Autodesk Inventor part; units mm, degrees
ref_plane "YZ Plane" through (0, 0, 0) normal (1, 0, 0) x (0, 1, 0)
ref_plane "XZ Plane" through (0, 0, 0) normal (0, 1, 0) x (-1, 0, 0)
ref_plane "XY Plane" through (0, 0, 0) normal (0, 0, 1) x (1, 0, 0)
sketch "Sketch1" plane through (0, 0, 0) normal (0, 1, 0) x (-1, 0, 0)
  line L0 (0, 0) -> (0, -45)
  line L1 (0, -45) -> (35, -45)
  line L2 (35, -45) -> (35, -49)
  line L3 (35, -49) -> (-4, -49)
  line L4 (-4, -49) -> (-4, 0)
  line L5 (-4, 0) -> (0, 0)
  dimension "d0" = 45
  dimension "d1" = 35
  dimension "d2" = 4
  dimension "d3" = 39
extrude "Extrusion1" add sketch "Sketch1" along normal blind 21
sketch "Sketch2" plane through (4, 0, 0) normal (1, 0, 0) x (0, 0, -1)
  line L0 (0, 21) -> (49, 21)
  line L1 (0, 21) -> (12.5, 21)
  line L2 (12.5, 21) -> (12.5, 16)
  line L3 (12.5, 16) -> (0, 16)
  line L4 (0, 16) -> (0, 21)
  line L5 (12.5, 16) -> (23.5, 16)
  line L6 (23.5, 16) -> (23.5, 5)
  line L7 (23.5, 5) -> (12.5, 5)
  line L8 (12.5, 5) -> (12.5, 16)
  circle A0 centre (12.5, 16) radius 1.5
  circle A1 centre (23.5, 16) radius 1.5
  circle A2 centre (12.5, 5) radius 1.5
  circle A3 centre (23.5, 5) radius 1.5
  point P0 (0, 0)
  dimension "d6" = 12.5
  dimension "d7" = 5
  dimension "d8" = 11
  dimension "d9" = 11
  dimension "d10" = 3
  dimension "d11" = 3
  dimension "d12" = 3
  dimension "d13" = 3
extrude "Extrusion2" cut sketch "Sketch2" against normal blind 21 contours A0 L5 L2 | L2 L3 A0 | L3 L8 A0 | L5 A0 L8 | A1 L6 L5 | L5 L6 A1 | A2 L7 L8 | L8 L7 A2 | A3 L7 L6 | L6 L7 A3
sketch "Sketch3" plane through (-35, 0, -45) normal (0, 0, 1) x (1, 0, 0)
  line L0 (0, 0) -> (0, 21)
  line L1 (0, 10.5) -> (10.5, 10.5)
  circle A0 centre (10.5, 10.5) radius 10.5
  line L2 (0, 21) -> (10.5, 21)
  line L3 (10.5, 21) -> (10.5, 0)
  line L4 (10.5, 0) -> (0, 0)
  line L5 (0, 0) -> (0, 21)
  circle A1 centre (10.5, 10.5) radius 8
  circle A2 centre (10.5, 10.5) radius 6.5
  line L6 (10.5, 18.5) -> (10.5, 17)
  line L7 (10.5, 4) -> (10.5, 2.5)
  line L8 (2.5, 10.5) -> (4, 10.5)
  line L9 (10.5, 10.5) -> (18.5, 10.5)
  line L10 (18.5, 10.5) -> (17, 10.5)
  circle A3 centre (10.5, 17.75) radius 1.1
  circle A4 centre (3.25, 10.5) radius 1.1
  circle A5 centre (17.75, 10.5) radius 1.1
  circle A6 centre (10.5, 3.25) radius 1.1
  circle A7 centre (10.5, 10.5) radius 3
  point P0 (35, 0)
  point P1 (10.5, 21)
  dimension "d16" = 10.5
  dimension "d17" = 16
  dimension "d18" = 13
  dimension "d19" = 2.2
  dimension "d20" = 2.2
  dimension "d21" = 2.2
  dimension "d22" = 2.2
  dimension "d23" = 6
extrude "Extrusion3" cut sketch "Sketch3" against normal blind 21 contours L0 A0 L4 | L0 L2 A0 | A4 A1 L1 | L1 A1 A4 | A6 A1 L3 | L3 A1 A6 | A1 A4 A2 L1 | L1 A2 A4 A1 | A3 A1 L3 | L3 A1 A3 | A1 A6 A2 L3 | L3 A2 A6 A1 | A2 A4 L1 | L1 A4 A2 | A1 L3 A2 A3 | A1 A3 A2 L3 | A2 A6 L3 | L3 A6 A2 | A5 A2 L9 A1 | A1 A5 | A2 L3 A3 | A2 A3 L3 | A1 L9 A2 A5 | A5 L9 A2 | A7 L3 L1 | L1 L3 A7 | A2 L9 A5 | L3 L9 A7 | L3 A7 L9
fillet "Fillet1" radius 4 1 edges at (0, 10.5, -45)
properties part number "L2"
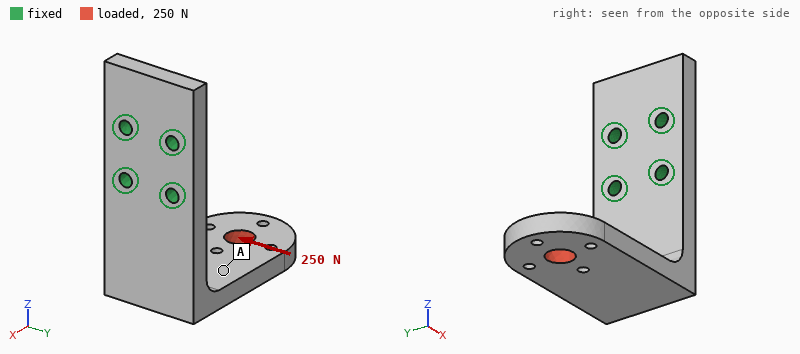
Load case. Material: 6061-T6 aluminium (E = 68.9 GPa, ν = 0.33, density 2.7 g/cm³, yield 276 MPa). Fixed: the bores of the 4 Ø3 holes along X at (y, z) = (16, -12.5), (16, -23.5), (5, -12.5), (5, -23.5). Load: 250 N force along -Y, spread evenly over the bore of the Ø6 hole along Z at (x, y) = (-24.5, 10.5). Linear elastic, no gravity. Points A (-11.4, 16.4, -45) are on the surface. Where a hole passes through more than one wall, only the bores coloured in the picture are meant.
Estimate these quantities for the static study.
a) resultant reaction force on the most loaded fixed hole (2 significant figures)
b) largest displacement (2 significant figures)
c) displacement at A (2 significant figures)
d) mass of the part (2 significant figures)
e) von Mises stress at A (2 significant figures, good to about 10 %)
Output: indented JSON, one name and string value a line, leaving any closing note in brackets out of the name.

{
  "resultant reaction force on the most loaded fixed hole": "620 N",
  "largest displacement": "0.35 mm",
  "displacement at A": "0.14 mm",
  "mass of the part": "18 g",
  "von Mises stress at A": "14 MPa"
}
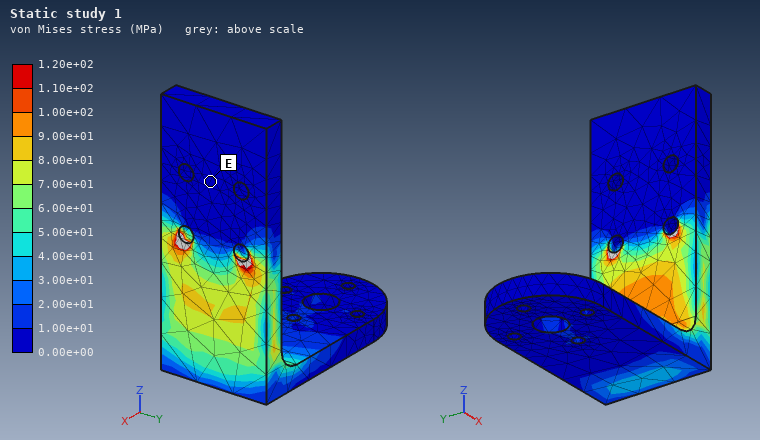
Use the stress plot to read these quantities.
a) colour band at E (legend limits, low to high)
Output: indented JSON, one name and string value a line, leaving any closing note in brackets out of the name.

{
  "colour band at E": "0.00e+00 to 1.00e+01 MPa"
}
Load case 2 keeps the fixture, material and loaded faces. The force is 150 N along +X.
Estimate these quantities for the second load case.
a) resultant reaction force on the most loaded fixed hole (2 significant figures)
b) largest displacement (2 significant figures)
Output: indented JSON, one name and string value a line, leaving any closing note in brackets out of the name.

{
  "resultant reaction force on the most loaded fixed hole": "110 N",
  "largest displacement": "0.20 mm"
}
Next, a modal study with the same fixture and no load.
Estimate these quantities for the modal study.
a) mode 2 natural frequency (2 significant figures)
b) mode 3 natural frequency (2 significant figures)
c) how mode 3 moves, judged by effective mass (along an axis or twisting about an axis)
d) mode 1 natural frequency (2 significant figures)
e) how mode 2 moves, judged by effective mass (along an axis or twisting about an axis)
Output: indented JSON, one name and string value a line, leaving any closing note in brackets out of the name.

{
  "mode 2 natural frequency": "2300 Hz",
  "mode 3 natural frequency": "4200 Hz",
  "how mode 3 moves, judged by effective mass": "along X",
  "mode 1 natural frequency": "1400 Hz",
  "how mode 2 moves, judged by effective mass": "along Y"
}
